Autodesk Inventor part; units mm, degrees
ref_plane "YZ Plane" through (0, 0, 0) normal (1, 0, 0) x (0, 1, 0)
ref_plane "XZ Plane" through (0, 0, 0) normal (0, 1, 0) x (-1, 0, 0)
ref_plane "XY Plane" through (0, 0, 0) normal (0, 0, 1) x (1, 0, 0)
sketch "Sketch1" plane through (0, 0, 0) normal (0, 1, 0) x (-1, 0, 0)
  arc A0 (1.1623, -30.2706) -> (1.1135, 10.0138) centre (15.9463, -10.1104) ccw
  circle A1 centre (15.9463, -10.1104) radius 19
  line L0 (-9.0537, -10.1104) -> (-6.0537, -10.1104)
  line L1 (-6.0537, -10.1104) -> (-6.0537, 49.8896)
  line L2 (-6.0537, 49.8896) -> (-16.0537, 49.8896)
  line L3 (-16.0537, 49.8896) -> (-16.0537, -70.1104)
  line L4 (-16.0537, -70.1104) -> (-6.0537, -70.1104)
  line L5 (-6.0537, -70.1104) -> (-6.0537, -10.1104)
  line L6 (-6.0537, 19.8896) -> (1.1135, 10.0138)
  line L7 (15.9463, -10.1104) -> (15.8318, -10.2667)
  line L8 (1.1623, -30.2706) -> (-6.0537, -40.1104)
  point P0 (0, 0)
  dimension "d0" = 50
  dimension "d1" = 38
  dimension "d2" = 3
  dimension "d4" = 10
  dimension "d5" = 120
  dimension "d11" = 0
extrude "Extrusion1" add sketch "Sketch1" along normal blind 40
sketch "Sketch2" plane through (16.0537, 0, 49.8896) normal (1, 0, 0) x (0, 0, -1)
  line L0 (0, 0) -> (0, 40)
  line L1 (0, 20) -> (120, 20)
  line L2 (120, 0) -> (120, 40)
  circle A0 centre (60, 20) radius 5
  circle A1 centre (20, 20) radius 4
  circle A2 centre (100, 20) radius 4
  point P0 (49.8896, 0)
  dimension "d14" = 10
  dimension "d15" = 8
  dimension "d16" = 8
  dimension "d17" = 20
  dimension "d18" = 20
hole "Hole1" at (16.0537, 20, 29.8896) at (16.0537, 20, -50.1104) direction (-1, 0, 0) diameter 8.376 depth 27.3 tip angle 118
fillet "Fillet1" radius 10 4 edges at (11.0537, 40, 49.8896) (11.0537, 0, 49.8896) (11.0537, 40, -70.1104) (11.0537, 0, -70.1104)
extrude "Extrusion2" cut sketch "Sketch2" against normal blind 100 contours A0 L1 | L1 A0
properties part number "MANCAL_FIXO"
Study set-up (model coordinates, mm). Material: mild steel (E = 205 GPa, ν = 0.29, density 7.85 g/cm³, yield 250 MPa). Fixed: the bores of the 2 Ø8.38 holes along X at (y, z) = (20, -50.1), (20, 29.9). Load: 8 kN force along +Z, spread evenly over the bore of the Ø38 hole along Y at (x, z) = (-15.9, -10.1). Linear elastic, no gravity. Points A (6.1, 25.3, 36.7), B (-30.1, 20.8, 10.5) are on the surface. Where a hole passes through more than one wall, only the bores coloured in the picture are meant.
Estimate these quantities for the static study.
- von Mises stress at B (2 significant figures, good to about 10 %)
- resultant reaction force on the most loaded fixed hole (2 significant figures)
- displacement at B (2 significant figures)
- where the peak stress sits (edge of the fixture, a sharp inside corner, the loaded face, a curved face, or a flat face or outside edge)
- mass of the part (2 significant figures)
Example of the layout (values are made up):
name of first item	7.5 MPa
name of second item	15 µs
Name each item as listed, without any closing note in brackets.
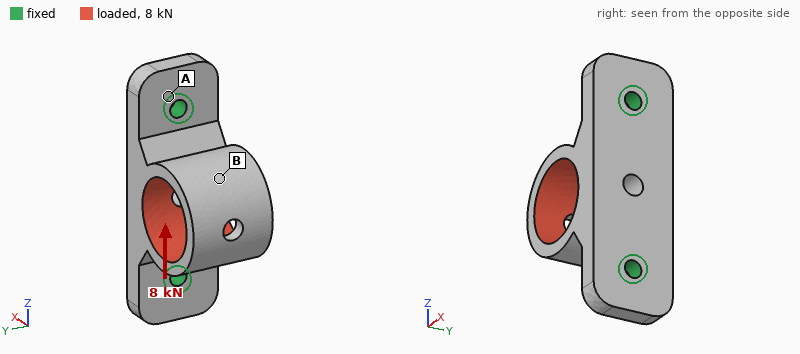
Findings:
von Mises stress at B	51 MPa
resultant reaction force on the most loaded fixed hole	5.1 kN
displacement at B	58 µm
where the peak stress sits	the loaded face
mass of the part	630 g
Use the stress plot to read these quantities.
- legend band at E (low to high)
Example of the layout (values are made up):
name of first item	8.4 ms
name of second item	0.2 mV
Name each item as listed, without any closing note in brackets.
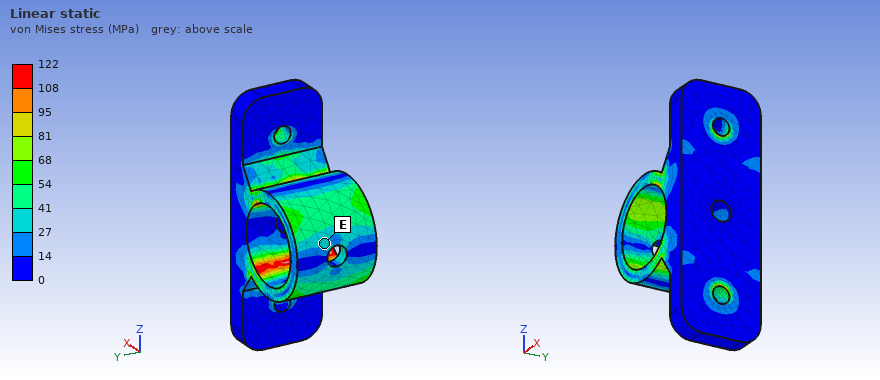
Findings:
legend band at E	27 to 41 MPa
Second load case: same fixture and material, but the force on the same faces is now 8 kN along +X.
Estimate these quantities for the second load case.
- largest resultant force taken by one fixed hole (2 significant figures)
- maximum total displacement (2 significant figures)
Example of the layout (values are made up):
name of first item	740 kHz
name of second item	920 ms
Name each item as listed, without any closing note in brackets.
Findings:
largest resultant force taken by one fixed hole	4.5 kN
maximum total displacement	15 µm
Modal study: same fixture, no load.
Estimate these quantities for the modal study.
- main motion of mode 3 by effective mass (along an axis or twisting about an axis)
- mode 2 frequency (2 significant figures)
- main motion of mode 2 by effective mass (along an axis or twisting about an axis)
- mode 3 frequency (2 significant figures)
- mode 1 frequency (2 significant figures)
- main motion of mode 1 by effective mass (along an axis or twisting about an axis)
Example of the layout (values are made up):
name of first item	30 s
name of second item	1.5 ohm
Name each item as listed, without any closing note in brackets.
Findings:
main motion of mode 3 by effective mass	along X
mode 2 frequency	3900 Hz
main motion of mode 2 by effective mass	along Z
mode 3 frequency	6200 Hz
mode 1 frequency	3000 Hz
main motion of mode 1 by effective mass	along Y
